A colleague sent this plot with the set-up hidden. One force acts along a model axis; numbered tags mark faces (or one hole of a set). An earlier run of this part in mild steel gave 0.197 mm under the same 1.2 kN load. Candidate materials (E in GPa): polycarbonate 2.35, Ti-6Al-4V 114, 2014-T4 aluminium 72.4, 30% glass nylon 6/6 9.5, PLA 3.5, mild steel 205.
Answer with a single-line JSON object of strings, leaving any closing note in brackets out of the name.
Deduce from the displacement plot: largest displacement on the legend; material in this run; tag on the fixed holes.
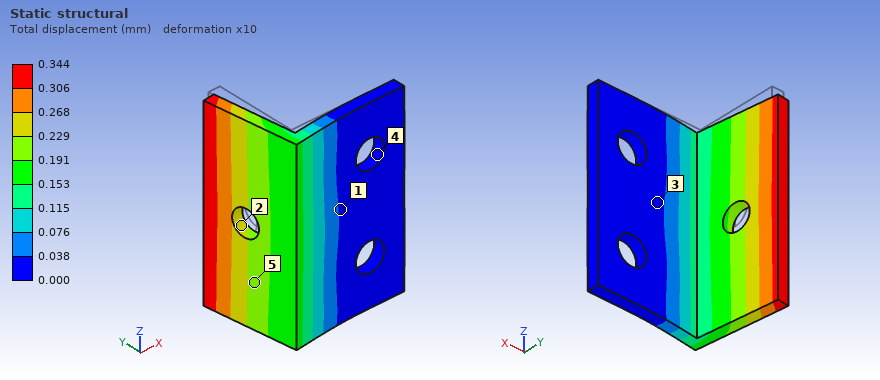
{"largest displacement on the legend": "0.344 mm", "material in this run": "Ti-6Al-4V", "tag on the fixed holes": "4"}
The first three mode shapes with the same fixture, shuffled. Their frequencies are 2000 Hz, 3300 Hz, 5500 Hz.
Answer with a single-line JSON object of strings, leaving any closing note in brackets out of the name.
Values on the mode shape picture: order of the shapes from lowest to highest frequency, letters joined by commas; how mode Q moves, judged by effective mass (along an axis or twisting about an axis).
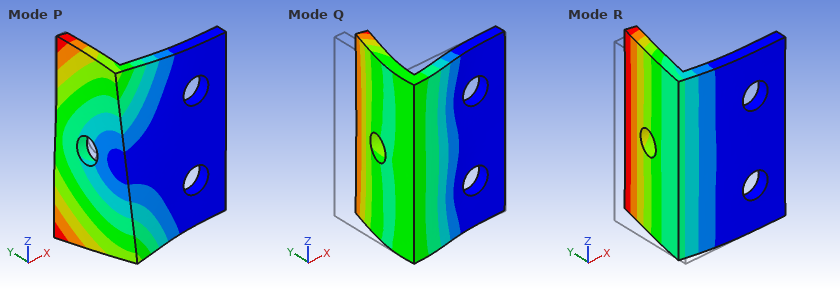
{"order of the shapes from lowest to highest frequency, letters joined by commas": "R, P, Q", "how mode Q moves, judged by effective mass": "along Y"}
